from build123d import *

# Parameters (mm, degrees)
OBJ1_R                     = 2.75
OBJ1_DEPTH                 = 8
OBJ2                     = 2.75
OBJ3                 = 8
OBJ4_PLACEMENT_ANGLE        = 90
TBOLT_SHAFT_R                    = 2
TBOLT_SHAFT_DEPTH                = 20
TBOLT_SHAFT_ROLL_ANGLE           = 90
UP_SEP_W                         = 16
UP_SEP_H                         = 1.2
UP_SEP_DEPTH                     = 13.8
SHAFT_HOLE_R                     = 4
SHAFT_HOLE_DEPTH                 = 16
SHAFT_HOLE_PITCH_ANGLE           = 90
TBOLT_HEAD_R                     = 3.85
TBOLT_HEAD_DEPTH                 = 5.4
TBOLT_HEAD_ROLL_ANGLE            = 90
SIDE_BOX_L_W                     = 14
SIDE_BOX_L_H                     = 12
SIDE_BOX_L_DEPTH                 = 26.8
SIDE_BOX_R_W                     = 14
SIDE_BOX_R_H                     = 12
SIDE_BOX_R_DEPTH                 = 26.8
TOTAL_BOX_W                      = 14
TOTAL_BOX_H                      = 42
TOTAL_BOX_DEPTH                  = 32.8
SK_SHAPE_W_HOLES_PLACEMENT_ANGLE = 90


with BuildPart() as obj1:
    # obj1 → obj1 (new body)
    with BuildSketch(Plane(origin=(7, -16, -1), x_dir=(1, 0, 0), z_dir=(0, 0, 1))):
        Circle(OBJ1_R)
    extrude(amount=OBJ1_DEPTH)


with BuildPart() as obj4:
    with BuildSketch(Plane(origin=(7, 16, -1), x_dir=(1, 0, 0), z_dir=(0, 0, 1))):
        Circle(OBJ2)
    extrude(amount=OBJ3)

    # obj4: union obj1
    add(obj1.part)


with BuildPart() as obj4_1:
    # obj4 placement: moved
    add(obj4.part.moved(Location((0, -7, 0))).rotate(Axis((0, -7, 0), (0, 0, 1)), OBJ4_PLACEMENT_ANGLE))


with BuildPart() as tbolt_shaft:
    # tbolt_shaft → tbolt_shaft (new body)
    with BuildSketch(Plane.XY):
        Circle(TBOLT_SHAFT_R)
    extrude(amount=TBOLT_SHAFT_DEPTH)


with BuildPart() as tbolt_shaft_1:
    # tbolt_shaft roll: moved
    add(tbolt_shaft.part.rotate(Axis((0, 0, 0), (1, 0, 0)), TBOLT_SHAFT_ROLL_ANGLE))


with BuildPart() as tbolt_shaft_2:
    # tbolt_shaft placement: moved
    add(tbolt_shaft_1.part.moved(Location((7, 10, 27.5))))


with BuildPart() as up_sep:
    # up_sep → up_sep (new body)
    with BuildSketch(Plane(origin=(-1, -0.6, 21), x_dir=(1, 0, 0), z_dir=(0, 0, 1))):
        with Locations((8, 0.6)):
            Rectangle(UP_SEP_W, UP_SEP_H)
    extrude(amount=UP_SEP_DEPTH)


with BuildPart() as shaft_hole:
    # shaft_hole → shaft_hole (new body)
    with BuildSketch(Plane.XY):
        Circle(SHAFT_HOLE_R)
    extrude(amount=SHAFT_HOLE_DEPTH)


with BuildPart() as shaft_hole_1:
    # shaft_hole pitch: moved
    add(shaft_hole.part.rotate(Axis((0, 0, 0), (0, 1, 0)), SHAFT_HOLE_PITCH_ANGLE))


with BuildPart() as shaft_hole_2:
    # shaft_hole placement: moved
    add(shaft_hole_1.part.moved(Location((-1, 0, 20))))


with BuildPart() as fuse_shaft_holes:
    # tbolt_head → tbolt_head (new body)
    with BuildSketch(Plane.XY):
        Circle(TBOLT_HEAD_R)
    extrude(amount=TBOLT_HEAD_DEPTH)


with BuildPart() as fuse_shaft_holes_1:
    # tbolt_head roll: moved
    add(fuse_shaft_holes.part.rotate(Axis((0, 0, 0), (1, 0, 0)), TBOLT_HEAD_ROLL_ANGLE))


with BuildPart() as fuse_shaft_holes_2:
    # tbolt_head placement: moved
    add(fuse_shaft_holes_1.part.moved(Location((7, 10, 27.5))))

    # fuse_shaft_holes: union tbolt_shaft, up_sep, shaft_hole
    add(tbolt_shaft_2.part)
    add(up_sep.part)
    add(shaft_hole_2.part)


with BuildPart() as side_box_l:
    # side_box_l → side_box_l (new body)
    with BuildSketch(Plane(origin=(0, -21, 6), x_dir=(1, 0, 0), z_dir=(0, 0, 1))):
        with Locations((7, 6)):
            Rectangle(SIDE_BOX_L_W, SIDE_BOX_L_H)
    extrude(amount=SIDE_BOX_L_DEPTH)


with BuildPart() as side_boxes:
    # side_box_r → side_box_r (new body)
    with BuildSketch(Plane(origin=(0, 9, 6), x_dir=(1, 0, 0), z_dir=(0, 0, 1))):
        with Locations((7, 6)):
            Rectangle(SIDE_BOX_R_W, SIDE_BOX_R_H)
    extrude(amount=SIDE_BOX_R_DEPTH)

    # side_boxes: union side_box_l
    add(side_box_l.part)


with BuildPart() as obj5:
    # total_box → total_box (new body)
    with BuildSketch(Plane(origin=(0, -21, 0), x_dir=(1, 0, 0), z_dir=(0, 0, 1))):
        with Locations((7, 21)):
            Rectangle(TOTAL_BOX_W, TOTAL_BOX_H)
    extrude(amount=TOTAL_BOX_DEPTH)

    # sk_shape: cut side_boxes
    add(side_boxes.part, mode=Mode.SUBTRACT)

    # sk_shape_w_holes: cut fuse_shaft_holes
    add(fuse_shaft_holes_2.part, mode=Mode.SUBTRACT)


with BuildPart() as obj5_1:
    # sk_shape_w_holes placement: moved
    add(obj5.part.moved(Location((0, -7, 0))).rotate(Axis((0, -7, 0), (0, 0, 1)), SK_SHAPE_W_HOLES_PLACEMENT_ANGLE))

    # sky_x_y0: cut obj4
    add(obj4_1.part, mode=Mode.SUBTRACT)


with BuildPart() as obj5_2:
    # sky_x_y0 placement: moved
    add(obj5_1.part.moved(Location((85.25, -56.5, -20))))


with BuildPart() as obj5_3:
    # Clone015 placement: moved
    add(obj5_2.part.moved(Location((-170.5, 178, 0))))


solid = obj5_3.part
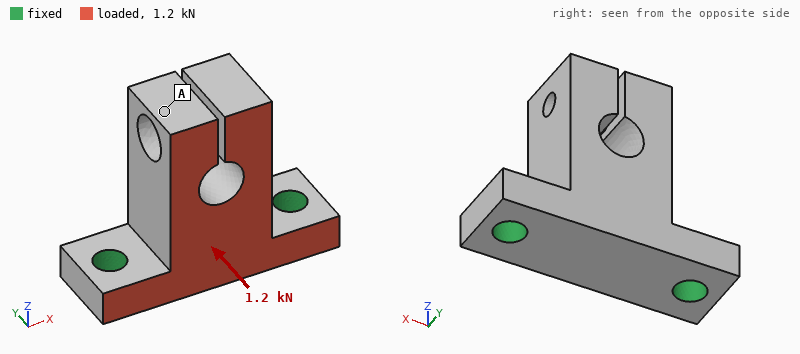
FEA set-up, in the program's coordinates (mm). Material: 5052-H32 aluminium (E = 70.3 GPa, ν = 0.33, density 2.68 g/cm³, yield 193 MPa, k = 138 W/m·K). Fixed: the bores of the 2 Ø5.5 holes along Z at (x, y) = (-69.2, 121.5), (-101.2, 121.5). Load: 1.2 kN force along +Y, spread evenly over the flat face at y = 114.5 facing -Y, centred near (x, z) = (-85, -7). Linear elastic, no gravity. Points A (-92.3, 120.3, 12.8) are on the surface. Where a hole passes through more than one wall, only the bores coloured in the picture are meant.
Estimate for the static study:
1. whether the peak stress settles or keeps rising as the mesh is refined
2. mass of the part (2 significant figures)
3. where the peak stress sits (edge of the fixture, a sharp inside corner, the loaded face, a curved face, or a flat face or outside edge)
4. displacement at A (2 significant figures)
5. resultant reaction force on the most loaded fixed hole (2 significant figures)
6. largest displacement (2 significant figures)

keeps rising
24 g
edge of the fixture
70 µm
600 N
72 µm
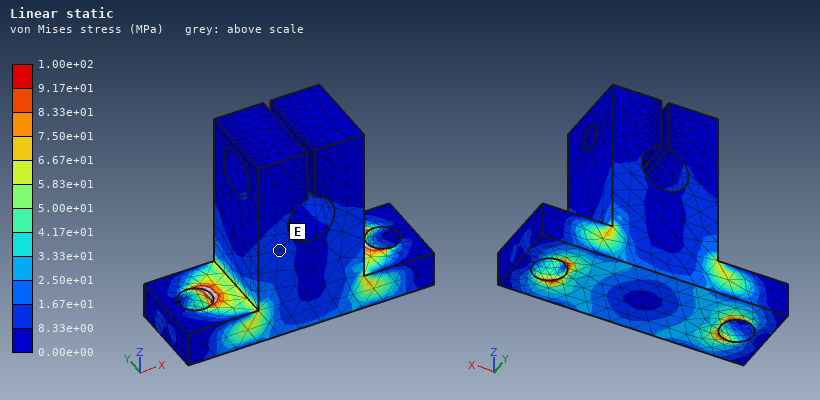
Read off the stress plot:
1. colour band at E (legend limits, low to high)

8.33e+00 to 1.67e+01 MPa
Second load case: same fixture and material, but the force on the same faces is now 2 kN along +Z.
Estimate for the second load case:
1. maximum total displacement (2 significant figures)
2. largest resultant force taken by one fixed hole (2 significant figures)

69 µm
1.0 kN
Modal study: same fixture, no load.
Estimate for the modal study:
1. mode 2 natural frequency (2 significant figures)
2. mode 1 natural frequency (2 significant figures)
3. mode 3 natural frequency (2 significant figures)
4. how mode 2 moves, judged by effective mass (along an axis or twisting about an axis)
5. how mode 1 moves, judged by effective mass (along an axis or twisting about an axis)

8500 Hz
5300 Hz
10 kHz
along X
along Y
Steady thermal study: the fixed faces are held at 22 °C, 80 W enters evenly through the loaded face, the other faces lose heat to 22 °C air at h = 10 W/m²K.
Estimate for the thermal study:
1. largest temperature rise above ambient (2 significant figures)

55 K
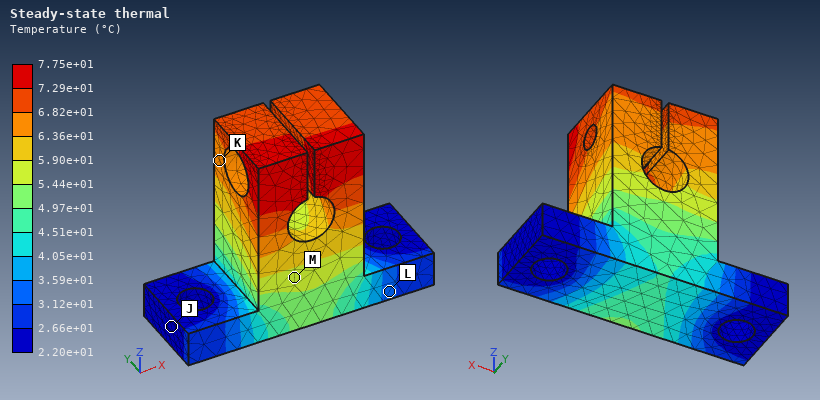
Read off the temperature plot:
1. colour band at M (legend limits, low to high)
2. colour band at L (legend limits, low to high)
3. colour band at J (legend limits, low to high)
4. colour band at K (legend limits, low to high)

5.44e+01 to 5.90e+01 °C
3.12e+01 to 3.59e+01 °C
2.20e+01 to 2.66e+01 °C
6.36e+01 to 6.82e+01 °C
